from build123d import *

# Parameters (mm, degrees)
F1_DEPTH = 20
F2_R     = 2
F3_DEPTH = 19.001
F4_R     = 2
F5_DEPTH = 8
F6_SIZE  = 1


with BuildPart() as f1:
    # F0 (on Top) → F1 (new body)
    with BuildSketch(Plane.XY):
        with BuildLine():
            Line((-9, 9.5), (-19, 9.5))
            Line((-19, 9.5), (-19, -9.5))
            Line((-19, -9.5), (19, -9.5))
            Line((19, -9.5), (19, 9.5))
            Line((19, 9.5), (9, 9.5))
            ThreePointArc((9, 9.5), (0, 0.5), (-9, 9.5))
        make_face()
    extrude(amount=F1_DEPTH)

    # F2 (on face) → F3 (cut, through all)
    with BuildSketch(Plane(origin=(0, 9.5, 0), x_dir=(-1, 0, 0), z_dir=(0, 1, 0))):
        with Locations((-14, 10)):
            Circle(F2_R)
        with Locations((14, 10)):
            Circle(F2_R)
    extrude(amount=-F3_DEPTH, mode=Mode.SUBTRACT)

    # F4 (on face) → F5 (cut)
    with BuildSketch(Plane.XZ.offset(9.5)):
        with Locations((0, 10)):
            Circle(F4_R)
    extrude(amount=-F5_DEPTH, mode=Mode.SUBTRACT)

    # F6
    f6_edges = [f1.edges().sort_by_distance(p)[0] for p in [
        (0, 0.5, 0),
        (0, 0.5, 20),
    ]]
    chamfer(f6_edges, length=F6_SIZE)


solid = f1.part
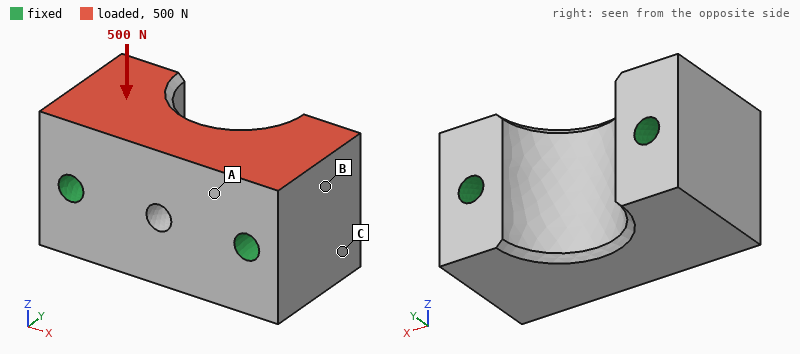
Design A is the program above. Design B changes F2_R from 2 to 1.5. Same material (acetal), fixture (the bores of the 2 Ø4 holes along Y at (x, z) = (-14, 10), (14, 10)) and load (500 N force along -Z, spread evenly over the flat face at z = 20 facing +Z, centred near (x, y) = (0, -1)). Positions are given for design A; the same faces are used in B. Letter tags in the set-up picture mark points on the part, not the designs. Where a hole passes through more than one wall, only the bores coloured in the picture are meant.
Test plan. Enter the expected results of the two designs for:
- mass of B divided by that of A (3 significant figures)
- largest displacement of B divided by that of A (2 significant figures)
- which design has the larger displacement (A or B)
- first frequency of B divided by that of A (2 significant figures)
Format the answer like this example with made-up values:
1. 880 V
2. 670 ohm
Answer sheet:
1. 1.02
2. 1.1
3. B
4. 0.91
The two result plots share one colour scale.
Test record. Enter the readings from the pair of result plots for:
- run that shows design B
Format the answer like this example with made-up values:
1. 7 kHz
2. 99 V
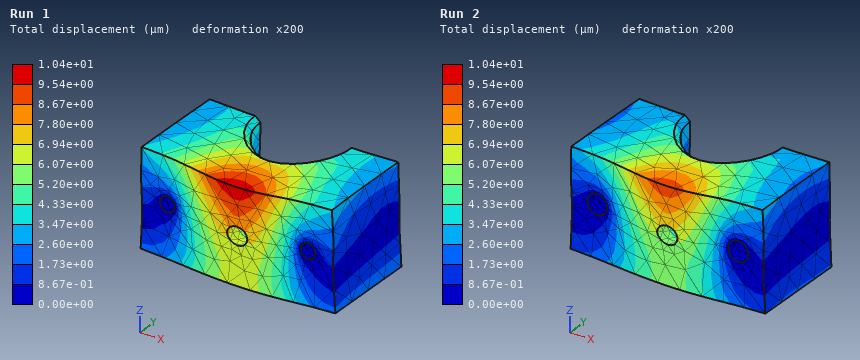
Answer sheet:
1. Run 1
